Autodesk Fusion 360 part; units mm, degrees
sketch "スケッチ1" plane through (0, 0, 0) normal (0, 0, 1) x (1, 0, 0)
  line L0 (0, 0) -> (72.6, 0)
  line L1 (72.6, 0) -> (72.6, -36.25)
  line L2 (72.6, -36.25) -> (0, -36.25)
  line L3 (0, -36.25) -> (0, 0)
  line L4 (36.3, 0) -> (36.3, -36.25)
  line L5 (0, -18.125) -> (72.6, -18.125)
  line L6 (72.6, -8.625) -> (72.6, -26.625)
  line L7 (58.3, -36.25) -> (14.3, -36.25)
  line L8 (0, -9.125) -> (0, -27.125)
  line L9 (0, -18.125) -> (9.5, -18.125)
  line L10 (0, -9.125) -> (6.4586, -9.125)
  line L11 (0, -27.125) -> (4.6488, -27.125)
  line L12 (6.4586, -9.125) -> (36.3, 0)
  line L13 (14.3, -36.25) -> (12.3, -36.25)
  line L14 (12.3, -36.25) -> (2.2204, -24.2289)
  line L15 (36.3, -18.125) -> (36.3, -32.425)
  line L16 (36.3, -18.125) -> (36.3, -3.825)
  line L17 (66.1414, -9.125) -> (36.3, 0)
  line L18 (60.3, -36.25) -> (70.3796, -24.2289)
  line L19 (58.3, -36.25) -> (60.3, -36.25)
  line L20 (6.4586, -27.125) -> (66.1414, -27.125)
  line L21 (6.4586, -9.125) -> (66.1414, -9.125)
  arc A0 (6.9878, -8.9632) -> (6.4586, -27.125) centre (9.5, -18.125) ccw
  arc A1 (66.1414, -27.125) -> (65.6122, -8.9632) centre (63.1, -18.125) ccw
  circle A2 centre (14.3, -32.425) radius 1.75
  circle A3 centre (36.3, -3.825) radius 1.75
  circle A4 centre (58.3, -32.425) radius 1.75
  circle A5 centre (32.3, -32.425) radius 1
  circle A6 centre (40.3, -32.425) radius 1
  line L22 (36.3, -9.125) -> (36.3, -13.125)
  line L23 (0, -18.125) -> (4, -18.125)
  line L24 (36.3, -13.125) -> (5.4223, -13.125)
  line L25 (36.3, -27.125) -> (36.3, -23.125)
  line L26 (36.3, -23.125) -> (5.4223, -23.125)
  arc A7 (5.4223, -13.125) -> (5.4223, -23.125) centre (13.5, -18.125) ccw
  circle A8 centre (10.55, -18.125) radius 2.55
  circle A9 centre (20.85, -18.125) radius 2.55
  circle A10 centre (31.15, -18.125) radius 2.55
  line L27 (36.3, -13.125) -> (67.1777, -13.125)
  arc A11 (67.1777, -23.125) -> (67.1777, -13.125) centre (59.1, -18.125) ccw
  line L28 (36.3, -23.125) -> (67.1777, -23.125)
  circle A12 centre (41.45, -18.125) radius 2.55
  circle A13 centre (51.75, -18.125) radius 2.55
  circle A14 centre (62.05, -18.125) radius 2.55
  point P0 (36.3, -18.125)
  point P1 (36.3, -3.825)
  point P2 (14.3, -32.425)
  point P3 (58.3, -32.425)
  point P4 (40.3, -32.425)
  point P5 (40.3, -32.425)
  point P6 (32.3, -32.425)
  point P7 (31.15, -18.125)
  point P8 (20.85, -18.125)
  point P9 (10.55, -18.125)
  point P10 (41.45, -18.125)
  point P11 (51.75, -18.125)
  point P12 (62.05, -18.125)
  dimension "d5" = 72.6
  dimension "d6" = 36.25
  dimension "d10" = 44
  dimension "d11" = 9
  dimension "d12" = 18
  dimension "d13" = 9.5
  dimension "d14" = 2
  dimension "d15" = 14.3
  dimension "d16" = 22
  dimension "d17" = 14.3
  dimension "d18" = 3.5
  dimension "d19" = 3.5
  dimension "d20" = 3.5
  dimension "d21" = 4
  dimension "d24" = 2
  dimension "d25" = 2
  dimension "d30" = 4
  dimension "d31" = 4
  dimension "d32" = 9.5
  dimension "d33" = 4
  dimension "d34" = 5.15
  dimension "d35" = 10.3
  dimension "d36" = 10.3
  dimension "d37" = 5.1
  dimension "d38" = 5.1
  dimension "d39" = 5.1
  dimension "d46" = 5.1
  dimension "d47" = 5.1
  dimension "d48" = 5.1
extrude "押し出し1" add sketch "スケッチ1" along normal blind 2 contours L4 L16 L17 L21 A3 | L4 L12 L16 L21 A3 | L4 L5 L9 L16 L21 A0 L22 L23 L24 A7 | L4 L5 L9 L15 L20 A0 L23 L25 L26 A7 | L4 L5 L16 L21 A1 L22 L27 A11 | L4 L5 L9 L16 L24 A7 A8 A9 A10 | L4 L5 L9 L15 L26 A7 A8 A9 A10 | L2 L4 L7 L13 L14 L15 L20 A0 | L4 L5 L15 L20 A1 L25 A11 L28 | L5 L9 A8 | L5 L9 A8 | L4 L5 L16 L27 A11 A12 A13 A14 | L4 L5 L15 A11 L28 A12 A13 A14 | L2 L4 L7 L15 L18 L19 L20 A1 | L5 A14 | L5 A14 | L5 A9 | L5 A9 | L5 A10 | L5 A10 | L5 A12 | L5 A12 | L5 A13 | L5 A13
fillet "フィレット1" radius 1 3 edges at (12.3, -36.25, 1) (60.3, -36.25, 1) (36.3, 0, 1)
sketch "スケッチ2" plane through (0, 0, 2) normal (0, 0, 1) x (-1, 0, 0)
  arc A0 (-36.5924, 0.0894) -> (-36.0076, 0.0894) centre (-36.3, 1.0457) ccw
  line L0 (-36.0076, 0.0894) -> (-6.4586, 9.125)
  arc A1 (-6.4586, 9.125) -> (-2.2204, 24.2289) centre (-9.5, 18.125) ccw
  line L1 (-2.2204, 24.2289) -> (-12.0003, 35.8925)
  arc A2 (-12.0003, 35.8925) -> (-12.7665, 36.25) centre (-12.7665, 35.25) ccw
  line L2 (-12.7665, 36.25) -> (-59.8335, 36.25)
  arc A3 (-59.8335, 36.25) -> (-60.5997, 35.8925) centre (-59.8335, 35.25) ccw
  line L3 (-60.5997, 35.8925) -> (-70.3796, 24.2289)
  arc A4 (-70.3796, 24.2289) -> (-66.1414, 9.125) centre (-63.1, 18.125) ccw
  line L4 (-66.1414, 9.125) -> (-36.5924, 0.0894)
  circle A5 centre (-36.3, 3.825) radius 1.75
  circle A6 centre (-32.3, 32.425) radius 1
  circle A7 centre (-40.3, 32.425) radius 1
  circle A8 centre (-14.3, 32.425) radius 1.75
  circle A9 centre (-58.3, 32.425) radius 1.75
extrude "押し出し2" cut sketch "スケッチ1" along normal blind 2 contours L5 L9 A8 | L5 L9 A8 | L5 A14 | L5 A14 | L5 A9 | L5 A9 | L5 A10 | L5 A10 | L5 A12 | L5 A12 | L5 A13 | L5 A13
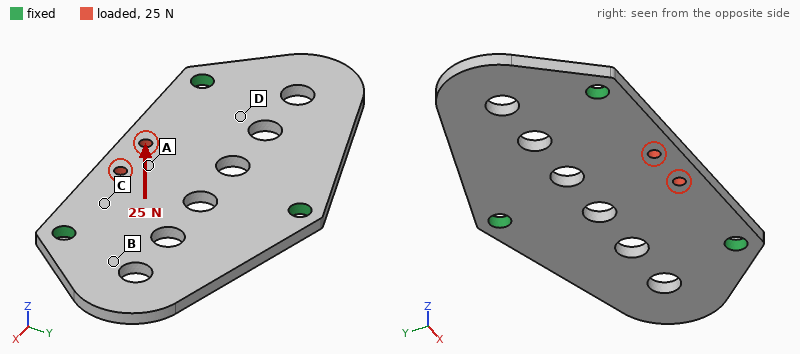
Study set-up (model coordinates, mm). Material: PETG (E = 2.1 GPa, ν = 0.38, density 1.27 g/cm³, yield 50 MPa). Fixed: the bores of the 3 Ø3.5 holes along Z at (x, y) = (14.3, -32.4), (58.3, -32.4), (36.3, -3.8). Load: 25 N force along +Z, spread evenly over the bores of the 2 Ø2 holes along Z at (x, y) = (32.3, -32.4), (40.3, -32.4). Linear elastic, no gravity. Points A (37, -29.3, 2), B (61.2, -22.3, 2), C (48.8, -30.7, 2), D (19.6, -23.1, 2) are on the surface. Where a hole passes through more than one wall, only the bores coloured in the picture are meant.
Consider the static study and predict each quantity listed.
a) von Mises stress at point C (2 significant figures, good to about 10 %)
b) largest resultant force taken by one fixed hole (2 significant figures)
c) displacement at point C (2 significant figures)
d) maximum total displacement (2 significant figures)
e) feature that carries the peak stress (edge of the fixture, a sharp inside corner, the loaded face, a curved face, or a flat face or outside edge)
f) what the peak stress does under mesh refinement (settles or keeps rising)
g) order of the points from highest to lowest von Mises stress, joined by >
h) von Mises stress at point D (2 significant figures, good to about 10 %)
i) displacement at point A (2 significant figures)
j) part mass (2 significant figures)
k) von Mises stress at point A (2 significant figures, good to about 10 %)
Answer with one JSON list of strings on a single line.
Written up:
["5.2 MPa", "11 N", "0.17 mm", "0.57 mm", "edge of the fixture", "keeps rising", "A > C > D > B", "3.1 MPa", "0.38 mm", "4.7 g", "6.7 MPa"]
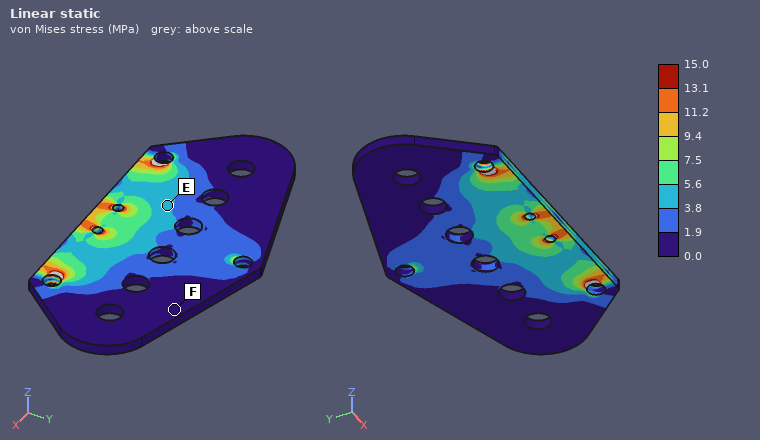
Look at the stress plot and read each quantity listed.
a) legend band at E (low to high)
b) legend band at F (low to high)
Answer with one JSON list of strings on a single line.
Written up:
["3.8 to 5.6 MPa", "0.0 to 1.9 MPa"]
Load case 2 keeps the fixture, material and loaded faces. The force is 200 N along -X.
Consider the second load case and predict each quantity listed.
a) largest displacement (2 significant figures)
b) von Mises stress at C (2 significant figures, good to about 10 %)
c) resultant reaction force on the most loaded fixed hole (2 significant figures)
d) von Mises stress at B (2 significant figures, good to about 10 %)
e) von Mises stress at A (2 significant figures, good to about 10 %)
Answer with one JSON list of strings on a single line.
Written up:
["51 µm", "4.3 MPa", "89 N", "1.3 MPa", "3.8 MPa"]
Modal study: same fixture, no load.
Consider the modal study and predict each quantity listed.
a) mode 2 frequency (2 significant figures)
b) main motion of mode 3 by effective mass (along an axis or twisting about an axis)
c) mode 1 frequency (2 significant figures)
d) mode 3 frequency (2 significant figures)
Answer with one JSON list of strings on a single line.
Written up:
["980 Hz", "along Z", "970 Hz", "1600 Hz"]
